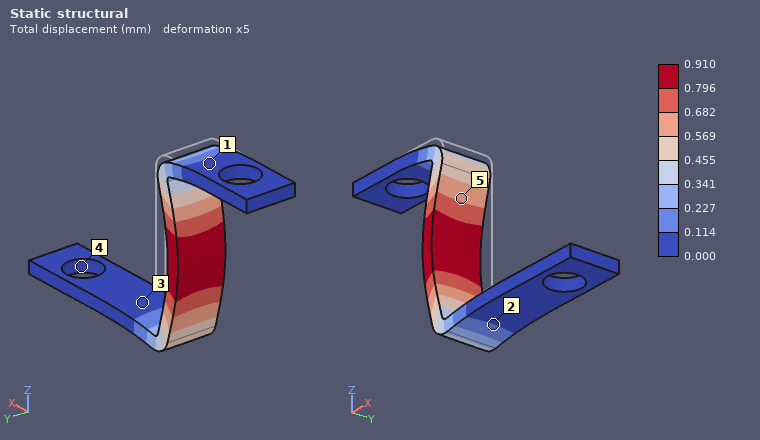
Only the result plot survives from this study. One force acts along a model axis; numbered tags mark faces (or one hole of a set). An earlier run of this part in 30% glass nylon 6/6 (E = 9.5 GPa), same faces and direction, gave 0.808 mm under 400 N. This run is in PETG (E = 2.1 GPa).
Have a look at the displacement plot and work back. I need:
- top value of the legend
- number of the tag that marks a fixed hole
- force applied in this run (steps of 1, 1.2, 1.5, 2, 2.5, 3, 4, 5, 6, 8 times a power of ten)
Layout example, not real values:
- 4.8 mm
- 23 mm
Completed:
- 0.910 mm
- 4
- 100 N
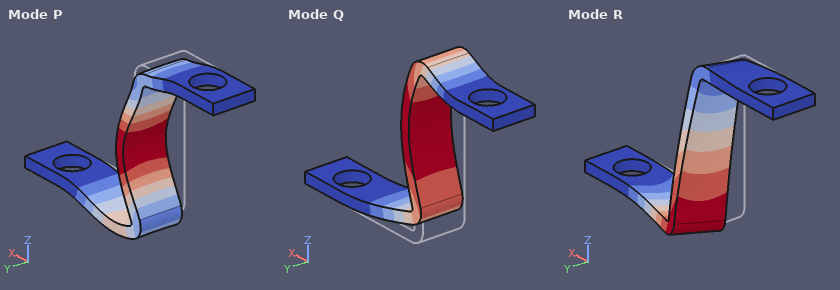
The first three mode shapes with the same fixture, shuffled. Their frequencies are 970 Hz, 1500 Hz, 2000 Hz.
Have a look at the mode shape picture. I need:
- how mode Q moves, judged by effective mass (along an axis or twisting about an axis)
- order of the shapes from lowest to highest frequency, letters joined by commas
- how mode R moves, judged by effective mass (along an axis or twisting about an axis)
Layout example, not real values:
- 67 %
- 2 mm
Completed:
- along Z
- Q, R, P
- along Y
